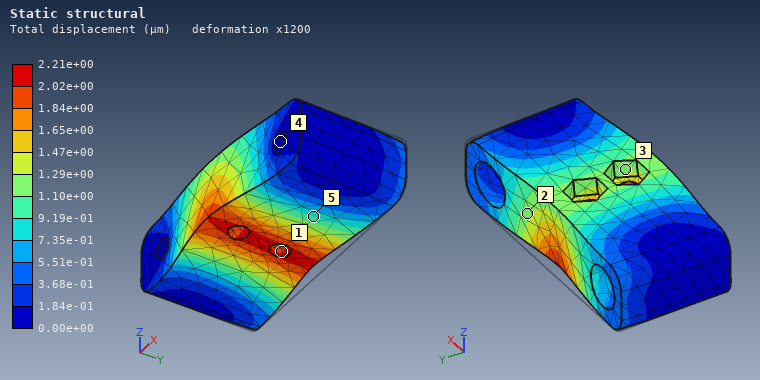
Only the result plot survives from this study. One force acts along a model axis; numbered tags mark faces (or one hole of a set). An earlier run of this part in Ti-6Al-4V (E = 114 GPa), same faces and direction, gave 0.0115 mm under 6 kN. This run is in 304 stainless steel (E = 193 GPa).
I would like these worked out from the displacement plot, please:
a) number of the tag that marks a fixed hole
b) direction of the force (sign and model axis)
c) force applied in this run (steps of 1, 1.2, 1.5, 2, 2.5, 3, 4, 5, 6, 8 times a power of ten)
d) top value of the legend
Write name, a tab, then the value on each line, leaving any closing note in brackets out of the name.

number of the tag that marks a fixed hole	4
direction of the force	-Y
force applied in this run	2 kN
top value of the legend	2.21e+00 µm
